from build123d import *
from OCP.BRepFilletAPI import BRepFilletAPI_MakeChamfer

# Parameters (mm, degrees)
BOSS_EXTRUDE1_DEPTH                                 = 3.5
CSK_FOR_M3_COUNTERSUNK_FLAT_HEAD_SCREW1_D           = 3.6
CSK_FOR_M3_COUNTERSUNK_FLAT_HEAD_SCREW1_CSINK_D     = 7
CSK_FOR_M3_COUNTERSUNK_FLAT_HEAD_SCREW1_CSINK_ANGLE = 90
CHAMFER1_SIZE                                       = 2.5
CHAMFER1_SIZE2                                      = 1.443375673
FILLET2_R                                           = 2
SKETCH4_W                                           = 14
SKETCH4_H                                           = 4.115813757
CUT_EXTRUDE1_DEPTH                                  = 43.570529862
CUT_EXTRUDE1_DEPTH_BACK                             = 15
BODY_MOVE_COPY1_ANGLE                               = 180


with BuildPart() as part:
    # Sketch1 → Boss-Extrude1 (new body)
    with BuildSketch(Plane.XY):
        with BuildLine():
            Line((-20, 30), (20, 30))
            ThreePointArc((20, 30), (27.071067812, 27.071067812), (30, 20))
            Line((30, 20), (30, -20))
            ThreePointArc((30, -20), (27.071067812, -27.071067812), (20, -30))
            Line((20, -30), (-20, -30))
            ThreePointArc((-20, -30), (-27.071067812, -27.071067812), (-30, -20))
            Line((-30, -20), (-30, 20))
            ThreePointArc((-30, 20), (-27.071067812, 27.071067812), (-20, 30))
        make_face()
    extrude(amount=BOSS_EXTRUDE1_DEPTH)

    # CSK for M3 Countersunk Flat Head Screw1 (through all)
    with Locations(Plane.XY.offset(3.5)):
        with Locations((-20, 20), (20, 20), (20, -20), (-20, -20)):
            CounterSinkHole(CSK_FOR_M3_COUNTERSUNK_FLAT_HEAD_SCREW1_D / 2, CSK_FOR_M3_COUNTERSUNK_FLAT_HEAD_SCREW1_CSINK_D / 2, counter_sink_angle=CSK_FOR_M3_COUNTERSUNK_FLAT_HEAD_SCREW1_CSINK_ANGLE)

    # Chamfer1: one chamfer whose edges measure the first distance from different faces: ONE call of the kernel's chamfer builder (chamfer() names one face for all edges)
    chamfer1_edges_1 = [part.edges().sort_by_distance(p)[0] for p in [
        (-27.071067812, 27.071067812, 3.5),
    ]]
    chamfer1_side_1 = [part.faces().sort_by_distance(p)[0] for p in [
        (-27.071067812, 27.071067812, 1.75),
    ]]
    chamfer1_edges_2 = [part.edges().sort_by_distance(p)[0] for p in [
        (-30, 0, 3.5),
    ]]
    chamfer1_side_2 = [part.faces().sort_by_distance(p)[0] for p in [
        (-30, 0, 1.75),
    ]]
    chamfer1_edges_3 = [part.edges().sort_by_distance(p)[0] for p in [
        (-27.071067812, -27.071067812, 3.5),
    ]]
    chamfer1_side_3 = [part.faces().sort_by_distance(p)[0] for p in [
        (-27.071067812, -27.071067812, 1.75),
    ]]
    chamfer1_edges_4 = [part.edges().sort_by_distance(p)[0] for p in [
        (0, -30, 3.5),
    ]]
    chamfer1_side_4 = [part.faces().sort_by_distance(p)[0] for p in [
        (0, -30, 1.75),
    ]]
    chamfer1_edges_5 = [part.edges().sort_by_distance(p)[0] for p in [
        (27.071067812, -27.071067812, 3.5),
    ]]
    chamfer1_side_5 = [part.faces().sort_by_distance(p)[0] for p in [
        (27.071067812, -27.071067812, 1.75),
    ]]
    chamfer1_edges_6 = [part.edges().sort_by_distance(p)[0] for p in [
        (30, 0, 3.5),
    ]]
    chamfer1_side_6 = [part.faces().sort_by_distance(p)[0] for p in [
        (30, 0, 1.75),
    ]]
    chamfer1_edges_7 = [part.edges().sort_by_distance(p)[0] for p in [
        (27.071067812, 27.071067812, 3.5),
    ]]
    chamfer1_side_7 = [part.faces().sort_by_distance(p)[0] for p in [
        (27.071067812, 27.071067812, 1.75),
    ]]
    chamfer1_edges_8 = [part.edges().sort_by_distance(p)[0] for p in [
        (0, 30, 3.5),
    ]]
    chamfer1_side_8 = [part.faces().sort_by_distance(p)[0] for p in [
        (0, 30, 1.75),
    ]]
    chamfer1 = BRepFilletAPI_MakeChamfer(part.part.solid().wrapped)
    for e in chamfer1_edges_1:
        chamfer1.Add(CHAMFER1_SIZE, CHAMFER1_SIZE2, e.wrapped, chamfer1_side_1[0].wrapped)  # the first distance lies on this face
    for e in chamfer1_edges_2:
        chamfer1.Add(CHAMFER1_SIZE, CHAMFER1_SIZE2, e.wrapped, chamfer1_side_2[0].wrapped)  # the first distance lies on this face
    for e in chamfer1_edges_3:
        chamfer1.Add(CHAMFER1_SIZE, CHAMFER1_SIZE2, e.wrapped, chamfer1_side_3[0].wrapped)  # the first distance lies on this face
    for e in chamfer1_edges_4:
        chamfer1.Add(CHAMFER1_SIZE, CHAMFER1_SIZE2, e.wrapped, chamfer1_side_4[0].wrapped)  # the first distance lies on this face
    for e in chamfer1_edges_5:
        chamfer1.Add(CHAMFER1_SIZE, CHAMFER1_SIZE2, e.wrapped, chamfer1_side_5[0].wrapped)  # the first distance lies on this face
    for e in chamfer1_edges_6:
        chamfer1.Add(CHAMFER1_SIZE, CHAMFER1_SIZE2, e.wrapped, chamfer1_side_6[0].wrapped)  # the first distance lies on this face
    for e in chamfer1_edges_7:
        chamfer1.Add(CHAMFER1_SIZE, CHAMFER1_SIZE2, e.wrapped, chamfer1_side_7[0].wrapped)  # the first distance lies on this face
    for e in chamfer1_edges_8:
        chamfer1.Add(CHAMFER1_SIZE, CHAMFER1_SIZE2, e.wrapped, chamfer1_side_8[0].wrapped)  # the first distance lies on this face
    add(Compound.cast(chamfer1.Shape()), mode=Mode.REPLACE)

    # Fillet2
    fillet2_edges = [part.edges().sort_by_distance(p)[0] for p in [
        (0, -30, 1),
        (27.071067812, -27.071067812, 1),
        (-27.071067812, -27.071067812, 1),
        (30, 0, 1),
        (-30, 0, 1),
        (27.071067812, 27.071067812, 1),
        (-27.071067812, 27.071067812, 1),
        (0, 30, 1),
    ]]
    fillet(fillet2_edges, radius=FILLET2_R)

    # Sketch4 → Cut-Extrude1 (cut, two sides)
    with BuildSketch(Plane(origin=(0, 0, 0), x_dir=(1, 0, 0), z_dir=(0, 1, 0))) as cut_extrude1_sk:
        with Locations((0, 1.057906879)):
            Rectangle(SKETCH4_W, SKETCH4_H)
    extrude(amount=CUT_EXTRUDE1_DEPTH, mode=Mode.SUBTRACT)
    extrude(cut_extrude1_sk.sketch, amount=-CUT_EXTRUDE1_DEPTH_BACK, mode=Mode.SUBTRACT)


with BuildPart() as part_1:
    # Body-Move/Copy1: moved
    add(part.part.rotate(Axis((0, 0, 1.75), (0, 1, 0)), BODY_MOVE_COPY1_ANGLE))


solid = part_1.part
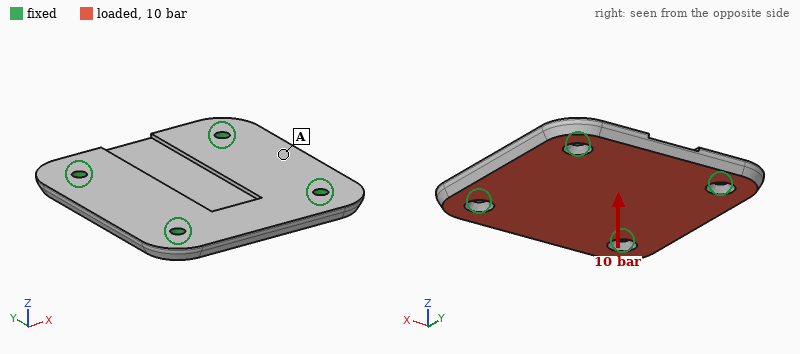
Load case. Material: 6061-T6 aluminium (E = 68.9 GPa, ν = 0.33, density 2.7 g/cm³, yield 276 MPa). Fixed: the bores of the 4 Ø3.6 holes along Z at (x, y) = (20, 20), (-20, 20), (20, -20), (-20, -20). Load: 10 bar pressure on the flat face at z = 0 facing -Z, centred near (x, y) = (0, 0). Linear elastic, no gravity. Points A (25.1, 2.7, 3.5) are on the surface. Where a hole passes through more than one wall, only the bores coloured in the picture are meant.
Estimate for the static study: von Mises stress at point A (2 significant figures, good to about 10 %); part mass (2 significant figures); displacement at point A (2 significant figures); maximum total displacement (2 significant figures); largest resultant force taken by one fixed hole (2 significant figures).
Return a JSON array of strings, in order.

["37 MPa", "30 g", "0.037 mm", "0.10 mm", "1.1 kN"]
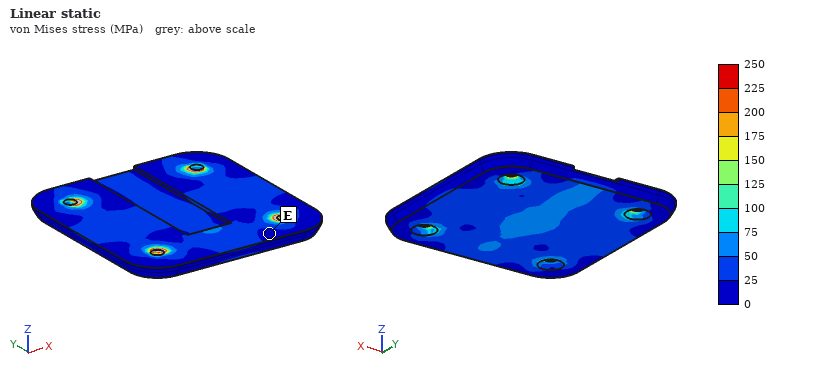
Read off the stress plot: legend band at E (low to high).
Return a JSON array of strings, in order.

["0 to 25 MPa"]
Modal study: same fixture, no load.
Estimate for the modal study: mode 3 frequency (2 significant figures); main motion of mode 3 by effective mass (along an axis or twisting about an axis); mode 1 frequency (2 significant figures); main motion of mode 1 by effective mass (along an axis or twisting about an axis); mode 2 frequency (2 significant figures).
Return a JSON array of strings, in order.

["9400 Hz", "twisting about Y", "6800 Hz", "along Z", "8700 Hz"]
